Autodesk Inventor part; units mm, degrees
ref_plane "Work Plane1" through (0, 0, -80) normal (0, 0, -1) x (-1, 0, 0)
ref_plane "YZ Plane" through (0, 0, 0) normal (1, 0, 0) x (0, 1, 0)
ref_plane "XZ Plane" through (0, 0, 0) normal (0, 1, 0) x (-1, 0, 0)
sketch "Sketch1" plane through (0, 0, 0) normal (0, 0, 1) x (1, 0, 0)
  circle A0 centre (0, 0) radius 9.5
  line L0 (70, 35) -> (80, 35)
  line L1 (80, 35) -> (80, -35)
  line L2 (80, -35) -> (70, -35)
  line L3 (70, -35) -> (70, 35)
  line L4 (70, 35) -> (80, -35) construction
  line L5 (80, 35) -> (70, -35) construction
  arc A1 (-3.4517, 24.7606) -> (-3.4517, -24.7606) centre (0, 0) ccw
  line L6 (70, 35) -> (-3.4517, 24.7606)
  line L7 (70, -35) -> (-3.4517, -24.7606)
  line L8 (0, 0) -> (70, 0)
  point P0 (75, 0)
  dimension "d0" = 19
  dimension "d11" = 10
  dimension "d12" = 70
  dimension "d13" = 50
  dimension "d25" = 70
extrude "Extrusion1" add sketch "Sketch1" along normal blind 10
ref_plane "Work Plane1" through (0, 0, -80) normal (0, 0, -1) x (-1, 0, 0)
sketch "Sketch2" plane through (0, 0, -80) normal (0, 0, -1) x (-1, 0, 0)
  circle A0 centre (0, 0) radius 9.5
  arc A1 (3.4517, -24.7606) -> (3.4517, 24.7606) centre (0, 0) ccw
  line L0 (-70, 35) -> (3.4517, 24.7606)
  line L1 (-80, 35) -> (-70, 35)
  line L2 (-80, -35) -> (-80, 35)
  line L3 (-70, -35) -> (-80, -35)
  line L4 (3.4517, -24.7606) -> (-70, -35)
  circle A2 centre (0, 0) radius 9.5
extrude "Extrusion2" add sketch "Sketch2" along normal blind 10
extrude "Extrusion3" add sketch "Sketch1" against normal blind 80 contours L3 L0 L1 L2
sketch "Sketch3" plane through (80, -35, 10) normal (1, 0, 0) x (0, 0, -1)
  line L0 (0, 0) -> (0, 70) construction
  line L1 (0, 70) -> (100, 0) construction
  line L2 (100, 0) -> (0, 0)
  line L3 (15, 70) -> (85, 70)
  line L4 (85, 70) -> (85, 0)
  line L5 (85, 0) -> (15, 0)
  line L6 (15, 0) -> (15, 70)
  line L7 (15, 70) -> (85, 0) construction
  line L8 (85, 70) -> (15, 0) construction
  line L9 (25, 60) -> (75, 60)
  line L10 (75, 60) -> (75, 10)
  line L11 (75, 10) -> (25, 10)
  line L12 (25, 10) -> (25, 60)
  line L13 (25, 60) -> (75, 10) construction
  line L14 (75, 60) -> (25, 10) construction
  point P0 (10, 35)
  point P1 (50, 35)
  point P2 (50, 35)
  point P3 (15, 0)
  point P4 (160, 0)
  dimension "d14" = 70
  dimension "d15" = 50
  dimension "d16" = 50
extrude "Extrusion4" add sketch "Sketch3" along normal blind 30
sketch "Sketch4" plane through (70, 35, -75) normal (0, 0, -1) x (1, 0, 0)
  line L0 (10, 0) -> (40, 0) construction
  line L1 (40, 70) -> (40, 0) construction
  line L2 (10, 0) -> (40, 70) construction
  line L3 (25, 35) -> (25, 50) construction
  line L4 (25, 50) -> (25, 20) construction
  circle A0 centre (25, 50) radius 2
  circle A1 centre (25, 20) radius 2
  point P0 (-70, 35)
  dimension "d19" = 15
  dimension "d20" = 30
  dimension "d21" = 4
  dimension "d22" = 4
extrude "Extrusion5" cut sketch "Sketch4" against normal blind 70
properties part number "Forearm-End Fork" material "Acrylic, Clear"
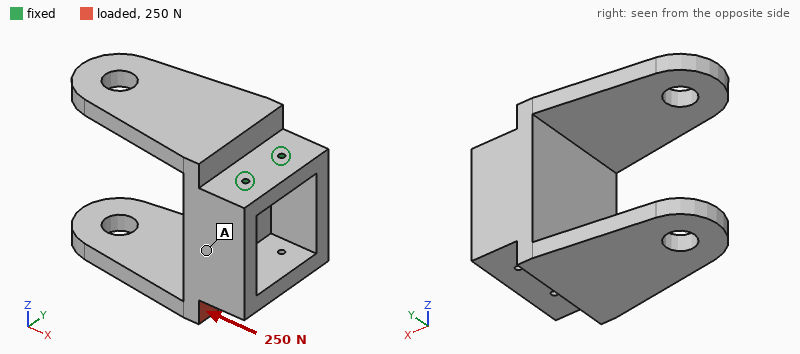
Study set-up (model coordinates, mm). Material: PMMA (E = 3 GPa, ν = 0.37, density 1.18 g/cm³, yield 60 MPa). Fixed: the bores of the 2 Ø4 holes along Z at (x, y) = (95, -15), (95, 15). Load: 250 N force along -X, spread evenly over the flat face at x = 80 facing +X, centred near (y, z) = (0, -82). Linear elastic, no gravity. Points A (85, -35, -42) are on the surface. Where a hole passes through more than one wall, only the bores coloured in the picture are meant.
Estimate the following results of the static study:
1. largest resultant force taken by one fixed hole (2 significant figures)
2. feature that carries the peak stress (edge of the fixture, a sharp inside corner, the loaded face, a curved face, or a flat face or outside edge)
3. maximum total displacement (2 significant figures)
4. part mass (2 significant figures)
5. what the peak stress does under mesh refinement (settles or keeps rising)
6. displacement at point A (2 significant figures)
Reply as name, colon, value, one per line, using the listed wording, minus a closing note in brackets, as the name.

largest resultant force taken by one fixed hole: 130 N
feature that carries the peak stress: edge of the fixture
maximum total displacement: 2.0 mm
part mass: 280 g
what the peak stress does under mesh refinement: keeps rising
displacement at point A: 0.41 mm
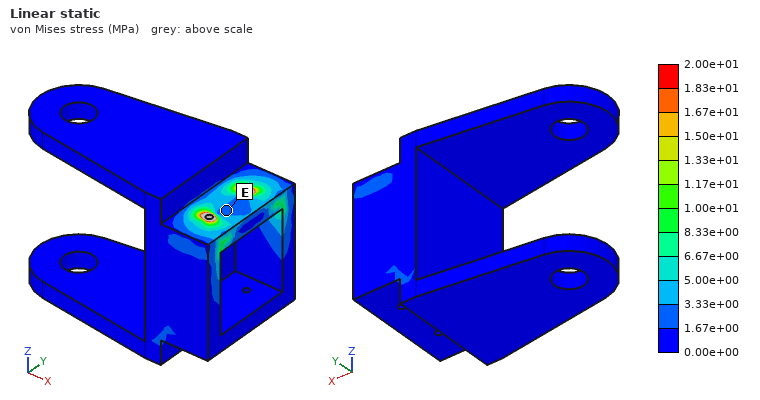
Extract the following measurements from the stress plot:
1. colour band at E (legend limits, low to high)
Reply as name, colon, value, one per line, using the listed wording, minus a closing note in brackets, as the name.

colour band at E: 1.67e+00 to 3.33e+00 MPa
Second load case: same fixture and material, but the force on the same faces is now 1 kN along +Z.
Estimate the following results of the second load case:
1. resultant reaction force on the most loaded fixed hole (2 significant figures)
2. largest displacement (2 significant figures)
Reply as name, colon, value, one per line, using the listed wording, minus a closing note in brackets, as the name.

resultant reaction force on the most loaded fixed hole: 500 N
largest displacement: 1.2 mm
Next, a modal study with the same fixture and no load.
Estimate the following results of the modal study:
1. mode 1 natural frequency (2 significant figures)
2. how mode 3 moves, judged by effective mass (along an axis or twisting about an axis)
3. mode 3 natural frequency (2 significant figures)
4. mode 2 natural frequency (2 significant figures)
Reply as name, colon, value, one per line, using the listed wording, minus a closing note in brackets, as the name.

mode 1 natural frequency: 160 Hz
how mode 3 moves, judged by effective mass: along X
mode 3 natural frequency: 420 Hz
mode 2 natural frequency: 280 Hz
